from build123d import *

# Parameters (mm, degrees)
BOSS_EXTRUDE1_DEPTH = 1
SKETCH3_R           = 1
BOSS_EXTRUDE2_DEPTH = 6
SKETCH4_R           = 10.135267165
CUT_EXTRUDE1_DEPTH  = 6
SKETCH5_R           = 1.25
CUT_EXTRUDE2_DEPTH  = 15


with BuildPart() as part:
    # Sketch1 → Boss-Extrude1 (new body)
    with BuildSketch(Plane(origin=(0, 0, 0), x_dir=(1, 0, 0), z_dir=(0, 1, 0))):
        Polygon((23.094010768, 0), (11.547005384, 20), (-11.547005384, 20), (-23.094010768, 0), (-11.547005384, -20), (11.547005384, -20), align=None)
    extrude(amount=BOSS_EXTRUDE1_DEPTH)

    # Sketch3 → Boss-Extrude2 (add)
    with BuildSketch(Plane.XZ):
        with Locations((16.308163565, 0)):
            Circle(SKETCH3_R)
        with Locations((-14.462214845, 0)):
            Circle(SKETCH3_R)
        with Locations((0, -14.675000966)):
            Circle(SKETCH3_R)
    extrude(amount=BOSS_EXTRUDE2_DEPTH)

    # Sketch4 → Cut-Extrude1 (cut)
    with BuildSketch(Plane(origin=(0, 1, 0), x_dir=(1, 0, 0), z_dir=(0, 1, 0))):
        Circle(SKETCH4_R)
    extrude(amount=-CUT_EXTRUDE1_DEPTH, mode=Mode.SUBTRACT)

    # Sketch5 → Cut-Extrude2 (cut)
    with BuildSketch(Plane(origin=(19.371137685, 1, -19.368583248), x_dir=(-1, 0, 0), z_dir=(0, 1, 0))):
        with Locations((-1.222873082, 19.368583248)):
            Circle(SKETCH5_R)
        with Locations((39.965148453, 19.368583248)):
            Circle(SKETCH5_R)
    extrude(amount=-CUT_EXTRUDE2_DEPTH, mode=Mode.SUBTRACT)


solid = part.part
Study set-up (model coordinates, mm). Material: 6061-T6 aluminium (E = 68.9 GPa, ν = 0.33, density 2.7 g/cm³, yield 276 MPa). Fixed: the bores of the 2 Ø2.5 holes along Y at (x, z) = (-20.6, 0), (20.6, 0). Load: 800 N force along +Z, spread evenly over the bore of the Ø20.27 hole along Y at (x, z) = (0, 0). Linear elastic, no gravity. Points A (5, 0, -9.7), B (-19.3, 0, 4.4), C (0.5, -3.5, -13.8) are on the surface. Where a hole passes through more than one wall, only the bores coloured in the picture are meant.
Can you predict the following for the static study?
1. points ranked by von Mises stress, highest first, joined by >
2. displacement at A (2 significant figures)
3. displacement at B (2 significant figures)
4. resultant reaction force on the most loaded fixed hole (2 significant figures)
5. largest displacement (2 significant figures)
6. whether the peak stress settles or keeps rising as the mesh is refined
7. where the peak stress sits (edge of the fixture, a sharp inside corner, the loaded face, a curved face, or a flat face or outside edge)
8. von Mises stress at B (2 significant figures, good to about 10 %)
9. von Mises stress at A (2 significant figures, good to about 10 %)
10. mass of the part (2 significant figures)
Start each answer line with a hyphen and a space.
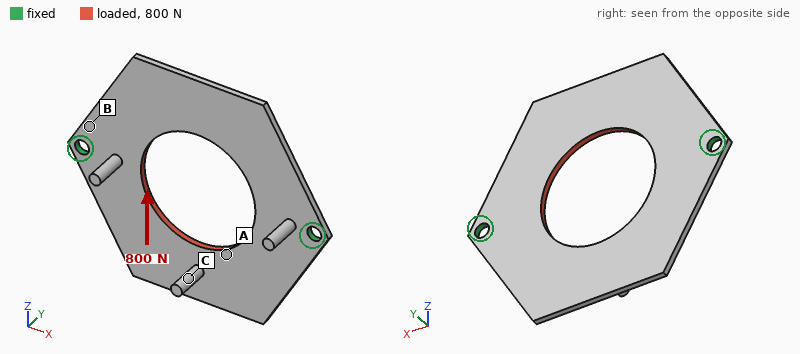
- B > A > C
- 14 µm
- 4.0 µm
- 400 N
- 14 µm
- keeps rising
- edge of the fixture
- 44 MPa
- 24 MPa
- 3.0 g
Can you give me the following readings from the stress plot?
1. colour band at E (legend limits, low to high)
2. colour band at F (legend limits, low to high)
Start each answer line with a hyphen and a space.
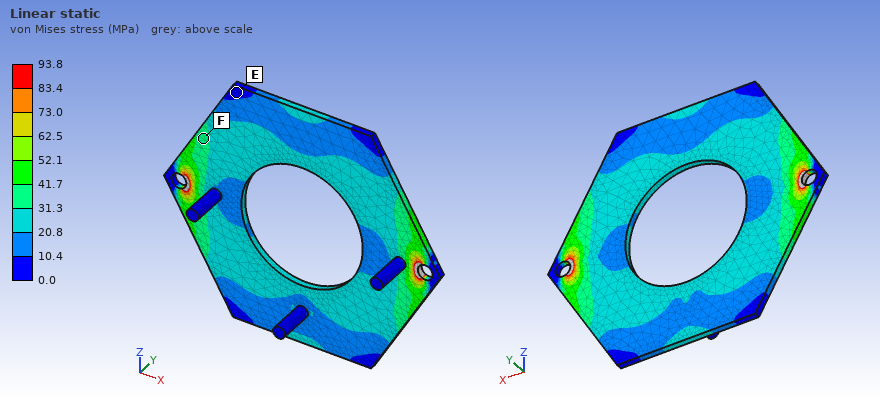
- 0.0 to 10.4 MPa
- 31.3 to 41.7 MPa
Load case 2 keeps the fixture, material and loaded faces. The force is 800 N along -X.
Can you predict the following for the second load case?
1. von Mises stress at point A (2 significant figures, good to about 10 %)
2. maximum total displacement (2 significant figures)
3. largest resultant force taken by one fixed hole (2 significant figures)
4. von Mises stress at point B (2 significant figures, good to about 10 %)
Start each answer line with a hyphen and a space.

- 26 MPa
- 12 µm
- 400 N
- 28 MPa
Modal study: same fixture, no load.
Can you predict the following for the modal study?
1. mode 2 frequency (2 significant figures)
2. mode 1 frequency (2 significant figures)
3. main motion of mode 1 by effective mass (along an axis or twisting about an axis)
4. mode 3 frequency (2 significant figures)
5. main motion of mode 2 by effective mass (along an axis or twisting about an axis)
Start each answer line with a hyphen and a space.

- 1600 Hz
- 1300 Hz
- twisting about X
- 3800 Hz
- along Y
